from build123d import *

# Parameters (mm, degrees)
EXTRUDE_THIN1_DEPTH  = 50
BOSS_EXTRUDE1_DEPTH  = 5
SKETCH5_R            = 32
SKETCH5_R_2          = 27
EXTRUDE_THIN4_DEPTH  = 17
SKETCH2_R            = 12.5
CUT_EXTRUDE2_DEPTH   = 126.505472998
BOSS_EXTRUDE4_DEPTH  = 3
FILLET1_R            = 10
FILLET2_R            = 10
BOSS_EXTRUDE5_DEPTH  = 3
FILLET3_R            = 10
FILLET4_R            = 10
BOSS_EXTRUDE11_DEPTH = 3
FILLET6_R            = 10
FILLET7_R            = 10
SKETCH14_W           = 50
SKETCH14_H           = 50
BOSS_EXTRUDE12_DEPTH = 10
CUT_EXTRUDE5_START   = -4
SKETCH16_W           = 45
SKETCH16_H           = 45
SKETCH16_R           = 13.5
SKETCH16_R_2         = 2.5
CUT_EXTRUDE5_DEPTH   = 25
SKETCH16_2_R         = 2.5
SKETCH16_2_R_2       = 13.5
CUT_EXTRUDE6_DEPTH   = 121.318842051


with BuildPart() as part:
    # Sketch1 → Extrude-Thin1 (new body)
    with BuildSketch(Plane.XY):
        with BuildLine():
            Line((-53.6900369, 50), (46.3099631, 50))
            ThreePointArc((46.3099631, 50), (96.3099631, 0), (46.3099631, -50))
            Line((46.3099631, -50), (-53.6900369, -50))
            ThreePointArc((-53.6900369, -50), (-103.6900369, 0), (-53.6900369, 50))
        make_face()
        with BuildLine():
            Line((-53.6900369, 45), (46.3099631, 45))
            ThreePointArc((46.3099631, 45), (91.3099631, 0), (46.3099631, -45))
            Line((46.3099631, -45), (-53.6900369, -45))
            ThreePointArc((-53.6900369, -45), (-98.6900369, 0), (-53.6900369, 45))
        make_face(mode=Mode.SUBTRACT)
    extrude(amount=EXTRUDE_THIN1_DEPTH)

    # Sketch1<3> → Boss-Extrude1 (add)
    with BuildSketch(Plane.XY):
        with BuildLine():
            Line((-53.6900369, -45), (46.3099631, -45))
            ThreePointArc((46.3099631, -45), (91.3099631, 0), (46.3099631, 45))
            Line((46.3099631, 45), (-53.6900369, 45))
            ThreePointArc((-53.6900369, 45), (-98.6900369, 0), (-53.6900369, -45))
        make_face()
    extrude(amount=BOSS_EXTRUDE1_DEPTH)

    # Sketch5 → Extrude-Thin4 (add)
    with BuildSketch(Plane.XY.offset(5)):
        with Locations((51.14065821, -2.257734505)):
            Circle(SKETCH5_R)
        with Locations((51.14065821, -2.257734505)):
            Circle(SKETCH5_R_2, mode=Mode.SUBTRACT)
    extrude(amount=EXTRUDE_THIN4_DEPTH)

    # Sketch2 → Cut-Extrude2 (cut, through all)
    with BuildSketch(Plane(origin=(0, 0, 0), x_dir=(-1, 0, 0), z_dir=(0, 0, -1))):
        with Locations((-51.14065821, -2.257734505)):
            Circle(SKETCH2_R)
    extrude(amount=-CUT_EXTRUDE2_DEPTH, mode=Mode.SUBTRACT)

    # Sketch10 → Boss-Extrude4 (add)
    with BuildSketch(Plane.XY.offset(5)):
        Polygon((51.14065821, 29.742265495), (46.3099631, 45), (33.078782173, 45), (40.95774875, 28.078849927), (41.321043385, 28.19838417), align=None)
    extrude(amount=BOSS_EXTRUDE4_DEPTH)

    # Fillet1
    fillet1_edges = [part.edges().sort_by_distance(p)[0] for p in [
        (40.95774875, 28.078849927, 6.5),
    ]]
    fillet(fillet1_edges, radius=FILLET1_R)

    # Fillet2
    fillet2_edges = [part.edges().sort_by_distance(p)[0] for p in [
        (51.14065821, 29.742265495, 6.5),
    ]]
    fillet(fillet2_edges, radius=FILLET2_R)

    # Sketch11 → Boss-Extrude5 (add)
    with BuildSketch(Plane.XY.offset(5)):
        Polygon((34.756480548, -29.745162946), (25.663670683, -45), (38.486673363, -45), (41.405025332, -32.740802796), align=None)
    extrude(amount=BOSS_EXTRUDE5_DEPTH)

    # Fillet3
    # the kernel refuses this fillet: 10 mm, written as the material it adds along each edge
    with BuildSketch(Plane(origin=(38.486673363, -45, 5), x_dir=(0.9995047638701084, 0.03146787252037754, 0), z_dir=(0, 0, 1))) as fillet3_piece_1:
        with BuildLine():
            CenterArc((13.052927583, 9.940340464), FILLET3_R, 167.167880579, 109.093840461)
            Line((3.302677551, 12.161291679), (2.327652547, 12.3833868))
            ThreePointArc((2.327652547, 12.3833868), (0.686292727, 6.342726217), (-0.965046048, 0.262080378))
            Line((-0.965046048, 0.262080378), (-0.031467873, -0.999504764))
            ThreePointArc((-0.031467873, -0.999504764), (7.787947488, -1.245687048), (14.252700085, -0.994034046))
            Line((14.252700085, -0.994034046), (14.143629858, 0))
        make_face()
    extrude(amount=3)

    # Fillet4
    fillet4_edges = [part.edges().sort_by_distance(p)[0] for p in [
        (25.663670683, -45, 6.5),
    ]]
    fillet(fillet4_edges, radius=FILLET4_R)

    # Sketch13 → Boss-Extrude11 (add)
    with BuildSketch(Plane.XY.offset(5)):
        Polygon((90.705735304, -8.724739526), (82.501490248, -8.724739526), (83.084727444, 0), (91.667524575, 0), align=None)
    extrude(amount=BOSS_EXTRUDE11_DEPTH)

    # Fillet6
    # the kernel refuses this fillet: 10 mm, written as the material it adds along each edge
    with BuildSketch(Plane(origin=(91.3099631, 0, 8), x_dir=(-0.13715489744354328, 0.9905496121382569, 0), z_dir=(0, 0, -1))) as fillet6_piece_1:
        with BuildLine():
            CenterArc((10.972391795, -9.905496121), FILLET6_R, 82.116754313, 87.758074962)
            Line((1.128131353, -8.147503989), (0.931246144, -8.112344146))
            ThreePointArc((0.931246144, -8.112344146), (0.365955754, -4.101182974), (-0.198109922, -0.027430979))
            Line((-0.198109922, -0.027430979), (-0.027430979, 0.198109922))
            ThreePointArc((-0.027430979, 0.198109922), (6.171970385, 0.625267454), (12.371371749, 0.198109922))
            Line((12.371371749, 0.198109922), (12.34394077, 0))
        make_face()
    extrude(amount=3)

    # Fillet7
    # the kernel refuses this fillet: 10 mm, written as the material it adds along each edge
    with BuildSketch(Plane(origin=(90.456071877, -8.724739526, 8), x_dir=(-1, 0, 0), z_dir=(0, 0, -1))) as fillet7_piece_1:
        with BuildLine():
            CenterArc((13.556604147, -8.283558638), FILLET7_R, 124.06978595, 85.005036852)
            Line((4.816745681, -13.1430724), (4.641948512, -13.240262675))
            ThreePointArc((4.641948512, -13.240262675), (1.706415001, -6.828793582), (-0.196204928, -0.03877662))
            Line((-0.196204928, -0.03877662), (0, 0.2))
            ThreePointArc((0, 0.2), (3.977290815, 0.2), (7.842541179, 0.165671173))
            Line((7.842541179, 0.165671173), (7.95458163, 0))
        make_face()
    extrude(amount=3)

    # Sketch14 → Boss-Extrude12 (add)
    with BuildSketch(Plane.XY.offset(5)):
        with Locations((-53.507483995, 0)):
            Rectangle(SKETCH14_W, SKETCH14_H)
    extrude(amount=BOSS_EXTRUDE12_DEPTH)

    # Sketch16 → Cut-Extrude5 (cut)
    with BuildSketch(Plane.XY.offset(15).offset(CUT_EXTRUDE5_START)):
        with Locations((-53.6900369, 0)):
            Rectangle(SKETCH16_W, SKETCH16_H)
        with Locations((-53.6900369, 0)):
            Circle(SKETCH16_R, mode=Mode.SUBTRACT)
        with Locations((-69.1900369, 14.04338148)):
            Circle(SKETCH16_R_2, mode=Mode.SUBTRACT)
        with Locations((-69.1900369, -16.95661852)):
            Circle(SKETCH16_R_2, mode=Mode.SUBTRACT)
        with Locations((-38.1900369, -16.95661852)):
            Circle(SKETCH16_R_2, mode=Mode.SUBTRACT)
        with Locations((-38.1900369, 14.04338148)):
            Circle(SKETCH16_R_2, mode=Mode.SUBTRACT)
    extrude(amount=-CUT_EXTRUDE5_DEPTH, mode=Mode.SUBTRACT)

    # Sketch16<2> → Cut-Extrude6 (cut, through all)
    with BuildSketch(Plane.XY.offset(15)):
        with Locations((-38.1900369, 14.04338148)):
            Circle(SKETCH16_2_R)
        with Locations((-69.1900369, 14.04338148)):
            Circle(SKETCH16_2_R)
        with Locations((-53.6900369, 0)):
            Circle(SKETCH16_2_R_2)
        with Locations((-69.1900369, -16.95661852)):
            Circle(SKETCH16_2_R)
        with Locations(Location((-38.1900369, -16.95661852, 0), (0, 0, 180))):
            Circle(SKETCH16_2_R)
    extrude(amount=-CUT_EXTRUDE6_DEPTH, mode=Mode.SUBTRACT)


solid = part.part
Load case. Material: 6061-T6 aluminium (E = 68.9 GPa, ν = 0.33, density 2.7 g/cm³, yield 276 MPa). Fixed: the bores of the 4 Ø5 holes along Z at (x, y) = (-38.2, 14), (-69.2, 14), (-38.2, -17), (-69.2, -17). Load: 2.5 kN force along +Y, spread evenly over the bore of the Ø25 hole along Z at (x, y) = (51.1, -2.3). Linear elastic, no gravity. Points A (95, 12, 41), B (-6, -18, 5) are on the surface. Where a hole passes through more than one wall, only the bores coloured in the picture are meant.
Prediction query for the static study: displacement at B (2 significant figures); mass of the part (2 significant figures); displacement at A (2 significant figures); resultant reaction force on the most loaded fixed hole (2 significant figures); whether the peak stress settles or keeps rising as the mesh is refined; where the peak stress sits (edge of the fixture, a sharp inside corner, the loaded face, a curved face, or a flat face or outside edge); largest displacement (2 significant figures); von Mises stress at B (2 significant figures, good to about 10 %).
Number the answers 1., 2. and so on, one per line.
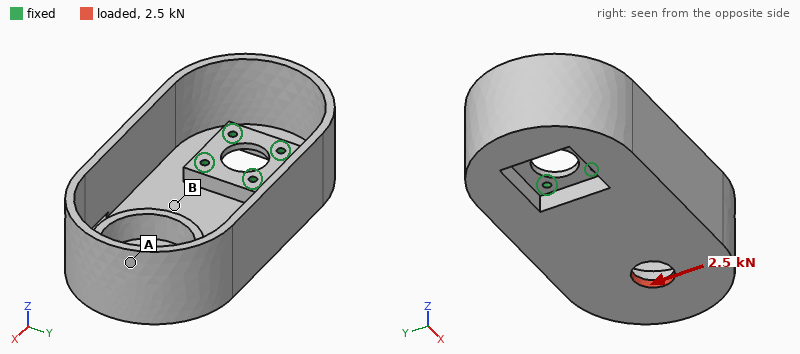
1. 0.048 mm
2. 580 g
3. 0.16 mm
4. 3.5 kN
5. keeps rising
6. edge of the fixture
7. 0.16 mm
8. 12 MPa
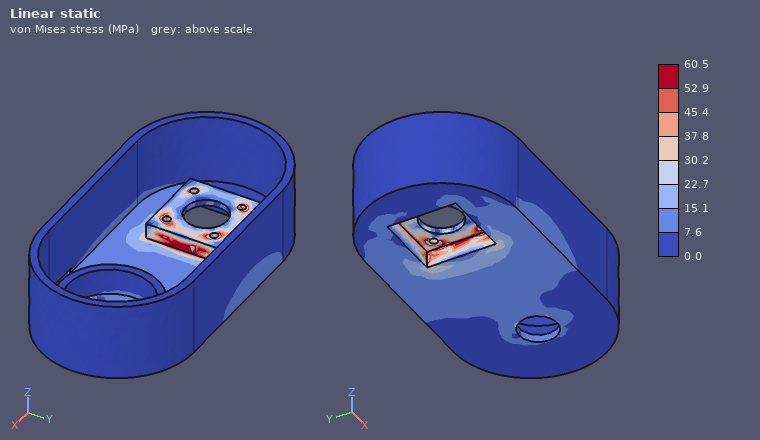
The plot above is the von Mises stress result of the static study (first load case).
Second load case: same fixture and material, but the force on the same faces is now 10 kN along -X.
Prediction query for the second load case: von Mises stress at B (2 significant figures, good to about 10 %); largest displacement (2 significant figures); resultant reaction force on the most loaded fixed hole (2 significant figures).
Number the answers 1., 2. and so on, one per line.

1. 25 MPa
2. 0.31 mm
3. 3.4 kN
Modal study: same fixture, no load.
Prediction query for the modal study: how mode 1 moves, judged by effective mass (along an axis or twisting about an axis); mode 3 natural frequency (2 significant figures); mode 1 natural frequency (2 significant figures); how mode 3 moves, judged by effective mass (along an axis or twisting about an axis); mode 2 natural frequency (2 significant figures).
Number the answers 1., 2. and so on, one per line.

1. along Z
2. 1300 Hz
3. 400 Hz
4. along Y
5. 670 Hz
